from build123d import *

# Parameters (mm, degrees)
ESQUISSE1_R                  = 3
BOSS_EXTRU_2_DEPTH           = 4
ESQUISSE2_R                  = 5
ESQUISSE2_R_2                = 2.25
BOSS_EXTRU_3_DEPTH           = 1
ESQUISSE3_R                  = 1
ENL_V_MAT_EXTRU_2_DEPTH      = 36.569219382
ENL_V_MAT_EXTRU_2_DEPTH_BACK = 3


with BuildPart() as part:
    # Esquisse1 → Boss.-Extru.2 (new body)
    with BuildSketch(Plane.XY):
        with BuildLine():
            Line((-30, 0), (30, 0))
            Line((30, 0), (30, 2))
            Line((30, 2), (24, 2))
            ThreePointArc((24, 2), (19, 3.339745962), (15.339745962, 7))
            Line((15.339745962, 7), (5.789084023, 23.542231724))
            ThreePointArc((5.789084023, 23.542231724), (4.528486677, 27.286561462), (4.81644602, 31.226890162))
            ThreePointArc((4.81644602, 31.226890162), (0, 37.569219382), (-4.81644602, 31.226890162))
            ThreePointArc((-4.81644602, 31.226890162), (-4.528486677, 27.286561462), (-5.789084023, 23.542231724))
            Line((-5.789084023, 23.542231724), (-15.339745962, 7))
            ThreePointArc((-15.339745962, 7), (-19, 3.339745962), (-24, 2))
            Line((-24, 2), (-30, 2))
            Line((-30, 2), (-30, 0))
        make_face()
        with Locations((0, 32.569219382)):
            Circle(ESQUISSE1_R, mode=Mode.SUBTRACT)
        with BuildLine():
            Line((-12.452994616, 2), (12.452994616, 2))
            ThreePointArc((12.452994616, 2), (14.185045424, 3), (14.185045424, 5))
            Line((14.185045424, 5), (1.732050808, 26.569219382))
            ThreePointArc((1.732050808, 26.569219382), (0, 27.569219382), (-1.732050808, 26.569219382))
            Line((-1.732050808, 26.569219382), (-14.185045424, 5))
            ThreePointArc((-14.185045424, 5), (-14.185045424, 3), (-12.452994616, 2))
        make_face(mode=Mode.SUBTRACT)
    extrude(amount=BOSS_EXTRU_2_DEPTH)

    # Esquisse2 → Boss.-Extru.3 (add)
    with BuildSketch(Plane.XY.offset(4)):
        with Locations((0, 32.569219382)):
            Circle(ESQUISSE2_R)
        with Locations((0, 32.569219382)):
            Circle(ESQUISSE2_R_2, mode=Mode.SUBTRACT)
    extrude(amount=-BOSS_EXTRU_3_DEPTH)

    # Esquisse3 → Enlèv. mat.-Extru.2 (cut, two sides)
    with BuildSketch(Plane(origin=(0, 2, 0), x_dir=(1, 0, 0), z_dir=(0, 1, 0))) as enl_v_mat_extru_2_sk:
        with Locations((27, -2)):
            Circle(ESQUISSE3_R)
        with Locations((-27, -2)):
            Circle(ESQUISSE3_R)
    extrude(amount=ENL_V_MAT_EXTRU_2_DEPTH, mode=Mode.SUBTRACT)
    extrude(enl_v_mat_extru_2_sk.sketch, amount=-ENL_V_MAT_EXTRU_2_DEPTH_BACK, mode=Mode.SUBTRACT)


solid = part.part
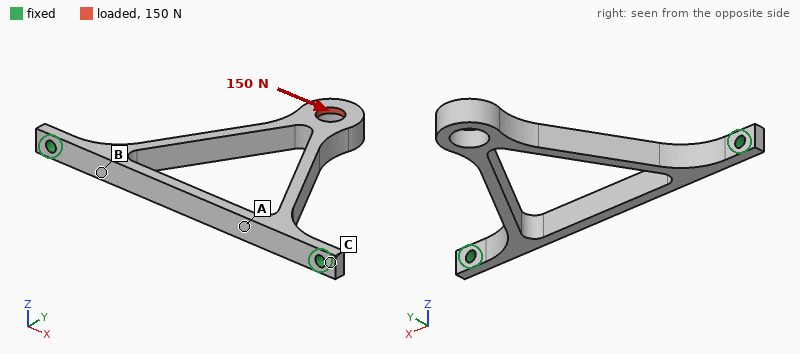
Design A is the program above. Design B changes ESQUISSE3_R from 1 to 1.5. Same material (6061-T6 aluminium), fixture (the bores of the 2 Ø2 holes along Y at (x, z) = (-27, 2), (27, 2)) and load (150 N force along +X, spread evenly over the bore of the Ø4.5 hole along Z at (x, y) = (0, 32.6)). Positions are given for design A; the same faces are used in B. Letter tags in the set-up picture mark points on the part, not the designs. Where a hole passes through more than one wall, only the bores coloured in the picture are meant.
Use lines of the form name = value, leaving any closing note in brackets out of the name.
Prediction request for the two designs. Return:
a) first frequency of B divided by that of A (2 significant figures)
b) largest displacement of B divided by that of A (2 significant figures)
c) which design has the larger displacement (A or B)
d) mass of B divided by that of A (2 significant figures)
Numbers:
first frequency of B divided by that of A = 1.0
largest displacement of B divided by that of A = 0.91
which design has the larger displacement = A
mass of B divided by that of A = 0.99
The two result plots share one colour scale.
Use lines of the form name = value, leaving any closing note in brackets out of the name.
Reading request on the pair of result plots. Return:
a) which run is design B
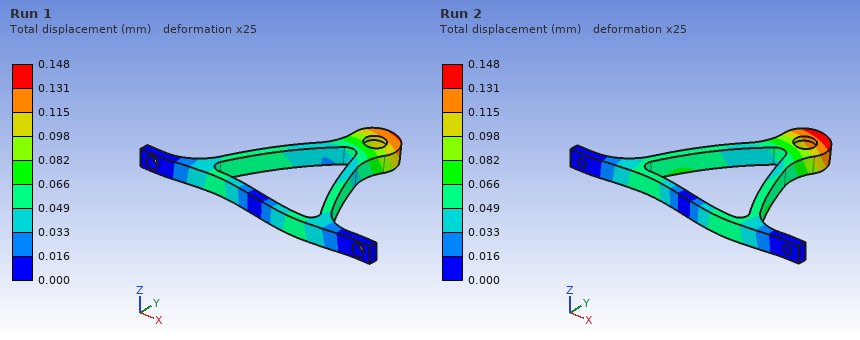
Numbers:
which run is design B = Run 1
